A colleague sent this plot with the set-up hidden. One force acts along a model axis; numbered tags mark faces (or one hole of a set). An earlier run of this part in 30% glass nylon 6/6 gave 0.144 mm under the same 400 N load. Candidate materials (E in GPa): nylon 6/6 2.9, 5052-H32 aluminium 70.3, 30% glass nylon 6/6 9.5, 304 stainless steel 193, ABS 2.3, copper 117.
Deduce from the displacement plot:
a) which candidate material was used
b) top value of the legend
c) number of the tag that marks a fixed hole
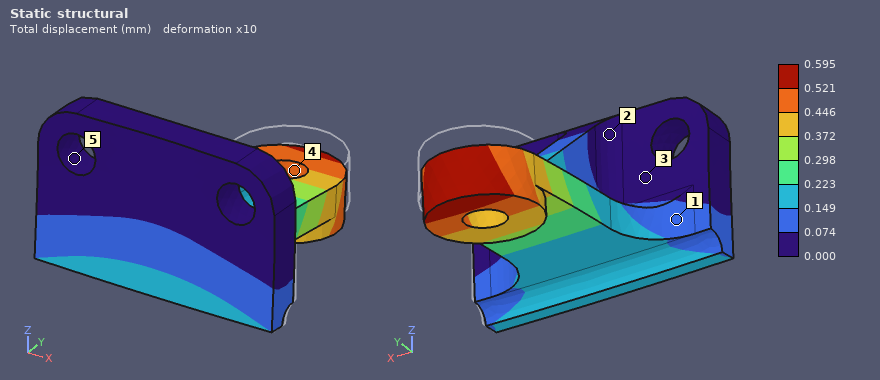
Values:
ABS
0.595 mm
5
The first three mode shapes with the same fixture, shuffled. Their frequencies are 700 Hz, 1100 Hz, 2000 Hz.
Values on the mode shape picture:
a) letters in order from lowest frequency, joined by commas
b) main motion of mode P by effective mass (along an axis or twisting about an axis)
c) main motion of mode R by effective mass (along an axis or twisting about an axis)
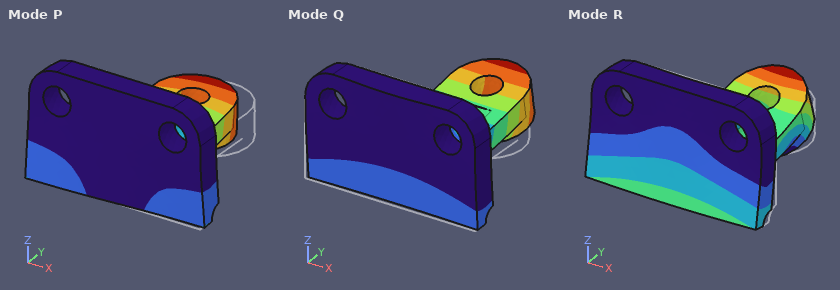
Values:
Q, P, R
along X
along Y
